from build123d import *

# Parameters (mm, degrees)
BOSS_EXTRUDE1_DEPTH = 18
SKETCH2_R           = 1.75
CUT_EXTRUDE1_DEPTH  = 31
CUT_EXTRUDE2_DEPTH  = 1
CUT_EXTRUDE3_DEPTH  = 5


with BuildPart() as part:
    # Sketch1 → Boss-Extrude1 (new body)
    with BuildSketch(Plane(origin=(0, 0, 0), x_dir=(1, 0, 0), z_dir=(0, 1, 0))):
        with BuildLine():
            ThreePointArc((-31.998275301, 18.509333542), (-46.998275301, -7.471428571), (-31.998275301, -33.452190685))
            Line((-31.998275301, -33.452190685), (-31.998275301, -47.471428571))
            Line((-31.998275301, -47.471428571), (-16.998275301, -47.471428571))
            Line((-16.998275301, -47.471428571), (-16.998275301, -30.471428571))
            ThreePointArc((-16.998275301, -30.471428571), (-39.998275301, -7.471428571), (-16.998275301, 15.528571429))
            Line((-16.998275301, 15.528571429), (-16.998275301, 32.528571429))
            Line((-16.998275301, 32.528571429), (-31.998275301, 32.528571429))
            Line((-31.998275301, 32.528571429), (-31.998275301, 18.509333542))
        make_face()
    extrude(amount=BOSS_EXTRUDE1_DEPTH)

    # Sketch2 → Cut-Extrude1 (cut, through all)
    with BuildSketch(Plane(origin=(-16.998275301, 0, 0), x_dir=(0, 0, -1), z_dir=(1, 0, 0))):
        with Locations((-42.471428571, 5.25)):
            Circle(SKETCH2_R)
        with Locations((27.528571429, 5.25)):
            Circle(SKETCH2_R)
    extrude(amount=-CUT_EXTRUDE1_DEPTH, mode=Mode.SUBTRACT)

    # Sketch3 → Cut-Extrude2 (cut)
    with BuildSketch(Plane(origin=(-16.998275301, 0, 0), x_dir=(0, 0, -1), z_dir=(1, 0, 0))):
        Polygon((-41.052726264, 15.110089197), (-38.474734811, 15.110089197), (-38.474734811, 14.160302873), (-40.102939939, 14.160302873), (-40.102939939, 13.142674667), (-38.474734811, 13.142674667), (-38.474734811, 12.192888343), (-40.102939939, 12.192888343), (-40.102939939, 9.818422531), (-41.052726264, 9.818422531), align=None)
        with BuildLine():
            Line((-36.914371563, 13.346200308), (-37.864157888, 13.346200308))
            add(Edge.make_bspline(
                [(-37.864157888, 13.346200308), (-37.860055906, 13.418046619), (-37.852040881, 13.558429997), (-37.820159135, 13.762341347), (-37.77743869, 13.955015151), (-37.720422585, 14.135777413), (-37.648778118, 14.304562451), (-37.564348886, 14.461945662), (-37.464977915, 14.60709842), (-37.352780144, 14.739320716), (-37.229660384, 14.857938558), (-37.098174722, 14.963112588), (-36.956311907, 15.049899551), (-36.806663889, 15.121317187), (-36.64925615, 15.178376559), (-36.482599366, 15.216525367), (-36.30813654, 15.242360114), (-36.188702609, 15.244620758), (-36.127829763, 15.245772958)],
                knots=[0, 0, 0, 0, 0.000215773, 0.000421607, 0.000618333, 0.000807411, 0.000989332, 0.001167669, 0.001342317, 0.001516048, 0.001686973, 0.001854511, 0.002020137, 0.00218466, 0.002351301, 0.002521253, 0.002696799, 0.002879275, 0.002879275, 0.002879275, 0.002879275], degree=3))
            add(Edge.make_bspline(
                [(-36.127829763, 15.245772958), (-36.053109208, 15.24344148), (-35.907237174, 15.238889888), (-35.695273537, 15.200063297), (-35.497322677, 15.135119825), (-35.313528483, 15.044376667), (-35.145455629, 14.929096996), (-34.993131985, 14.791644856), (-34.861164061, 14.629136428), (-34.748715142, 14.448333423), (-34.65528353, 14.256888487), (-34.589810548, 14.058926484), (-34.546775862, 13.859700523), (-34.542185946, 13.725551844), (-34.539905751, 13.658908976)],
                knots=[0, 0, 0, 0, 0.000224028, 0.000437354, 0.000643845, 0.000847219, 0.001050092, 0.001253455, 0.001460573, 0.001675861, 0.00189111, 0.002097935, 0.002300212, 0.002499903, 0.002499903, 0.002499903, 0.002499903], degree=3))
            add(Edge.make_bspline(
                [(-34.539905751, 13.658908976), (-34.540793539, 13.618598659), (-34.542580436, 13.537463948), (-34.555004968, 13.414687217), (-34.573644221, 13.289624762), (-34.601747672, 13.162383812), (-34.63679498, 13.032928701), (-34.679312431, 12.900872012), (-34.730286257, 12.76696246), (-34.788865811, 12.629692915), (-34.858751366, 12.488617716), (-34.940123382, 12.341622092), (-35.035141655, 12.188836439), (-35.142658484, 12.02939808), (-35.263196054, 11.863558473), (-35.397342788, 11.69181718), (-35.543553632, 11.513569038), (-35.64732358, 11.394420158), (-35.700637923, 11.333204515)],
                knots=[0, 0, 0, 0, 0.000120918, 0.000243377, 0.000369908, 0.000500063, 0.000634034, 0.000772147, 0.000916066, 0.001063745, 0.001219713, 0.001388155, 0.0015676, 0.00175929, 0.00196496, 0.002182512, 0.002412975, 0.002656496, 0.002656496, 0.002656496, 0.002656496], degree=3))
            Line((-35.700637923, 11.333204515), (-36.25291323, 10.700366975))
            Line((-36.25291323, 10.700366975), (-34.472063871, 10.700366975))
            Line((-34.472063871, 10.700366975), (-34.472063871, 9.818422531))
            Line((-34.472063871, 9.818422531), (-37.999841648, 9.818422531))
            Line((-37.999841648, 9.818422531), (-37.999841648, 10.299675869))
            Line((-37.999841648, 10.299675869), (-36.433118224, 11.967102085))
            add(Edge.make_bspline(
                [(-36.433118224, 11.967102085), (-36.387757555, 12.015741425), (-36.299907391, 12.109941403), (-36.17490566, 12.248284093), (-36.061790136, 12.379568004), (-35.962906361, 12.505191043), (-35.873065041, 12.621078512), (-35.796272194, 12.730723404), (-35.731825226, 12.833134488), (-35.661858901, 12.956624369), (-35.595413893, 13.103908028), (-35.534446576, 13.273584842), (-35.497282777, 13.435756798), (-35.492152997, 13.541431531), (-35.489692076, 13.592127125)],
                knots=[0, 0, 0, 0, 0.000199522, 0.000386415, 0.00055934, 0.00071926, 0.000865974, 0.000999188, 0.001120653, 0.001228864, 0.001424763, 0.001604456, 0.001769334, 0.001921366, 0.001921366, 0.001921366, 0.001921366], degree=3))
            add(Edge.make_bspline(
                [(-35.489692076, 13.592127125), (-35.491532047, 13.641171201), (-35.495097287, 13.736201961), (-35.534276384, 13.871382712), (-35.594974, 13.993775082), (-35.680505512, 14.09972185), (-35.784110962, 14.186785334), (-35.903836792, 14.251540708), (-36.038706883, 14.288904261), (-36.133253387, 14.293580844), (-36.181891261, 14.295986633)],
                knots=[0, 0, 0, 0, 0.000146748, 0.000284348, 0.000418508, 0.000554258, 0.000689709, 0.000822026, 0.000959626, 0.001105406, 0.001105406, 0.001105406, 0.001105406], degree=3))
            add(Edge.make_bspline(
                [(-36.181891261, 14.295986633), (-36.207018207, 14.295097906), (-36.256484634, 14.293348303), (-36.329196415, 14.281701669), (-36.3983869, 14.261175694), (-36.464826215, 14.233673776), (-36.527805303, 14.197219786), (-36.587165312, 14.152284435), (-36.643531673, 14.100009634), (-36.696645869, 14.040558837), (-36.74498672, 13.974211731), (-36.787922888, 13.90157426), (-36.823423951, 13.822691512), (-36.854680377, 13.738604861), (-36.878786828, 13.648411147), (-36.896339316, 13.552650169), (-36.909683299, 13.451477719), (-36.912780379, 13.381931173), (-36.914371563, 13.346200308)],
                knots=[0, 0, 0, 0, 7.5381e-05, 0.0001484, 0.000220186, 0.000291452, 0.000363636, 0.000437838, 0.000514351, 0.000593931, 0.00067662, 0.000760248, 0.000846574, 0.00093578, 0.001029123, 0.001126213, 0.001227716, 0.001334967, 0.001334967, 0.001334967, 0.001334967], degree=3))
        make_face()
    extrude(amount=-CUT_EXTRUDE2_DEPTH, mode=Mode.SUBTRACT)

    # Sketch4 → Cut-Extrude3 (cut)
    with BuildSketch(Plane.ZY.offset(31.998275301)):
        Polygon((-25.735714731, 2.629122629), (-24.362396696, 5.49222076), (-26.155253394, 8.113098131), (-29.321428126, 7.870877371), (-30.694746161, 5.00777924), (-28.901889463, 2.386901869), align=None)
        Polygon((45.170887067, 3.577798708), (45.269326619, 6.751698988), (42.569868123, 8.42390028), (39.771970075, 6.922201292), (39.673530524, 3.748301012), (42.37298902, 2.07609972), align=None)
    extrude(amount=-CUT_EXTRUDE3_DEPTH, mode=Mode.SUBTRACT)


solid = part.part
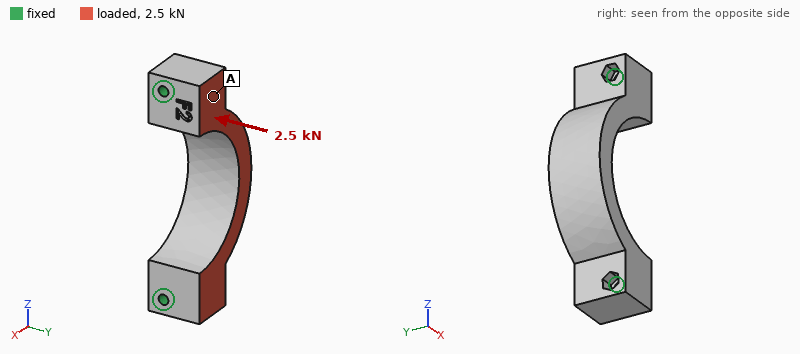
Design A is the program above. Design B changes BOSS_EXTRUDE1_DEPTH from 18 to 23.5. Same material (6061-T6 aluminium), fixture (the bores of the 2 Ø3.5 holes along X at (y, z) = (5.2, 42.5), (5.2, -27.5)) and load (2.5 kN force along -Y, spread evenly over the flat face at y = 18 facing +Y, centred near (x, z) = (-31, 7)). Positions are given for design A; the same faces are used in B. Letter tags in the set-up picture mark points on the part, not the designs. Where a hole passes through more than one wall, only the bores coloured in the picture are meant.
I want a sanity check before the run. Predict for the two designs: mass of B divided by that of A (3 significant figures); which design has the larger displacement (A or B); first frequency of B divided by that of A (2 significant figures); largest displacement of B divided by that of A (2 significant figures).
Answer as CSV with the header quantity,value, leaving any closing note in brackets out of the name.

quantity,value
mass of B divided by that of A,1.31
which design has the larger displacement,A
first frequency of B divided by that of A,0.90
largest displacement of B divided by that of A,0.91
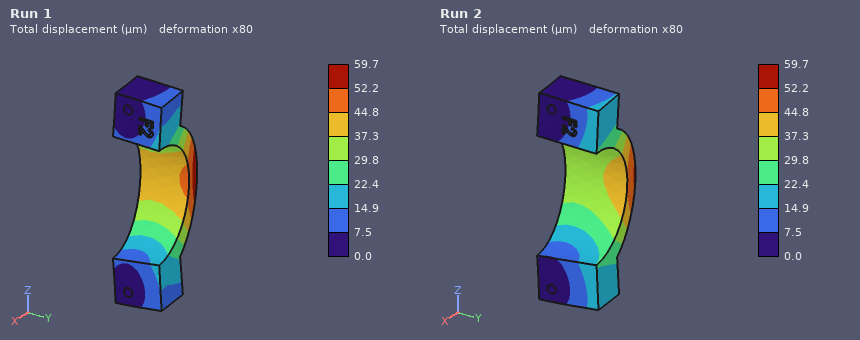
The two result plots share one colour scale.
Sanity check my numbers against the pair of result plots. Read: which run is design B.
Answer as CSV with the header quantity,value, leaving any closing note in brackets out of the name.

quantity,value
which run is design B,Run 2
